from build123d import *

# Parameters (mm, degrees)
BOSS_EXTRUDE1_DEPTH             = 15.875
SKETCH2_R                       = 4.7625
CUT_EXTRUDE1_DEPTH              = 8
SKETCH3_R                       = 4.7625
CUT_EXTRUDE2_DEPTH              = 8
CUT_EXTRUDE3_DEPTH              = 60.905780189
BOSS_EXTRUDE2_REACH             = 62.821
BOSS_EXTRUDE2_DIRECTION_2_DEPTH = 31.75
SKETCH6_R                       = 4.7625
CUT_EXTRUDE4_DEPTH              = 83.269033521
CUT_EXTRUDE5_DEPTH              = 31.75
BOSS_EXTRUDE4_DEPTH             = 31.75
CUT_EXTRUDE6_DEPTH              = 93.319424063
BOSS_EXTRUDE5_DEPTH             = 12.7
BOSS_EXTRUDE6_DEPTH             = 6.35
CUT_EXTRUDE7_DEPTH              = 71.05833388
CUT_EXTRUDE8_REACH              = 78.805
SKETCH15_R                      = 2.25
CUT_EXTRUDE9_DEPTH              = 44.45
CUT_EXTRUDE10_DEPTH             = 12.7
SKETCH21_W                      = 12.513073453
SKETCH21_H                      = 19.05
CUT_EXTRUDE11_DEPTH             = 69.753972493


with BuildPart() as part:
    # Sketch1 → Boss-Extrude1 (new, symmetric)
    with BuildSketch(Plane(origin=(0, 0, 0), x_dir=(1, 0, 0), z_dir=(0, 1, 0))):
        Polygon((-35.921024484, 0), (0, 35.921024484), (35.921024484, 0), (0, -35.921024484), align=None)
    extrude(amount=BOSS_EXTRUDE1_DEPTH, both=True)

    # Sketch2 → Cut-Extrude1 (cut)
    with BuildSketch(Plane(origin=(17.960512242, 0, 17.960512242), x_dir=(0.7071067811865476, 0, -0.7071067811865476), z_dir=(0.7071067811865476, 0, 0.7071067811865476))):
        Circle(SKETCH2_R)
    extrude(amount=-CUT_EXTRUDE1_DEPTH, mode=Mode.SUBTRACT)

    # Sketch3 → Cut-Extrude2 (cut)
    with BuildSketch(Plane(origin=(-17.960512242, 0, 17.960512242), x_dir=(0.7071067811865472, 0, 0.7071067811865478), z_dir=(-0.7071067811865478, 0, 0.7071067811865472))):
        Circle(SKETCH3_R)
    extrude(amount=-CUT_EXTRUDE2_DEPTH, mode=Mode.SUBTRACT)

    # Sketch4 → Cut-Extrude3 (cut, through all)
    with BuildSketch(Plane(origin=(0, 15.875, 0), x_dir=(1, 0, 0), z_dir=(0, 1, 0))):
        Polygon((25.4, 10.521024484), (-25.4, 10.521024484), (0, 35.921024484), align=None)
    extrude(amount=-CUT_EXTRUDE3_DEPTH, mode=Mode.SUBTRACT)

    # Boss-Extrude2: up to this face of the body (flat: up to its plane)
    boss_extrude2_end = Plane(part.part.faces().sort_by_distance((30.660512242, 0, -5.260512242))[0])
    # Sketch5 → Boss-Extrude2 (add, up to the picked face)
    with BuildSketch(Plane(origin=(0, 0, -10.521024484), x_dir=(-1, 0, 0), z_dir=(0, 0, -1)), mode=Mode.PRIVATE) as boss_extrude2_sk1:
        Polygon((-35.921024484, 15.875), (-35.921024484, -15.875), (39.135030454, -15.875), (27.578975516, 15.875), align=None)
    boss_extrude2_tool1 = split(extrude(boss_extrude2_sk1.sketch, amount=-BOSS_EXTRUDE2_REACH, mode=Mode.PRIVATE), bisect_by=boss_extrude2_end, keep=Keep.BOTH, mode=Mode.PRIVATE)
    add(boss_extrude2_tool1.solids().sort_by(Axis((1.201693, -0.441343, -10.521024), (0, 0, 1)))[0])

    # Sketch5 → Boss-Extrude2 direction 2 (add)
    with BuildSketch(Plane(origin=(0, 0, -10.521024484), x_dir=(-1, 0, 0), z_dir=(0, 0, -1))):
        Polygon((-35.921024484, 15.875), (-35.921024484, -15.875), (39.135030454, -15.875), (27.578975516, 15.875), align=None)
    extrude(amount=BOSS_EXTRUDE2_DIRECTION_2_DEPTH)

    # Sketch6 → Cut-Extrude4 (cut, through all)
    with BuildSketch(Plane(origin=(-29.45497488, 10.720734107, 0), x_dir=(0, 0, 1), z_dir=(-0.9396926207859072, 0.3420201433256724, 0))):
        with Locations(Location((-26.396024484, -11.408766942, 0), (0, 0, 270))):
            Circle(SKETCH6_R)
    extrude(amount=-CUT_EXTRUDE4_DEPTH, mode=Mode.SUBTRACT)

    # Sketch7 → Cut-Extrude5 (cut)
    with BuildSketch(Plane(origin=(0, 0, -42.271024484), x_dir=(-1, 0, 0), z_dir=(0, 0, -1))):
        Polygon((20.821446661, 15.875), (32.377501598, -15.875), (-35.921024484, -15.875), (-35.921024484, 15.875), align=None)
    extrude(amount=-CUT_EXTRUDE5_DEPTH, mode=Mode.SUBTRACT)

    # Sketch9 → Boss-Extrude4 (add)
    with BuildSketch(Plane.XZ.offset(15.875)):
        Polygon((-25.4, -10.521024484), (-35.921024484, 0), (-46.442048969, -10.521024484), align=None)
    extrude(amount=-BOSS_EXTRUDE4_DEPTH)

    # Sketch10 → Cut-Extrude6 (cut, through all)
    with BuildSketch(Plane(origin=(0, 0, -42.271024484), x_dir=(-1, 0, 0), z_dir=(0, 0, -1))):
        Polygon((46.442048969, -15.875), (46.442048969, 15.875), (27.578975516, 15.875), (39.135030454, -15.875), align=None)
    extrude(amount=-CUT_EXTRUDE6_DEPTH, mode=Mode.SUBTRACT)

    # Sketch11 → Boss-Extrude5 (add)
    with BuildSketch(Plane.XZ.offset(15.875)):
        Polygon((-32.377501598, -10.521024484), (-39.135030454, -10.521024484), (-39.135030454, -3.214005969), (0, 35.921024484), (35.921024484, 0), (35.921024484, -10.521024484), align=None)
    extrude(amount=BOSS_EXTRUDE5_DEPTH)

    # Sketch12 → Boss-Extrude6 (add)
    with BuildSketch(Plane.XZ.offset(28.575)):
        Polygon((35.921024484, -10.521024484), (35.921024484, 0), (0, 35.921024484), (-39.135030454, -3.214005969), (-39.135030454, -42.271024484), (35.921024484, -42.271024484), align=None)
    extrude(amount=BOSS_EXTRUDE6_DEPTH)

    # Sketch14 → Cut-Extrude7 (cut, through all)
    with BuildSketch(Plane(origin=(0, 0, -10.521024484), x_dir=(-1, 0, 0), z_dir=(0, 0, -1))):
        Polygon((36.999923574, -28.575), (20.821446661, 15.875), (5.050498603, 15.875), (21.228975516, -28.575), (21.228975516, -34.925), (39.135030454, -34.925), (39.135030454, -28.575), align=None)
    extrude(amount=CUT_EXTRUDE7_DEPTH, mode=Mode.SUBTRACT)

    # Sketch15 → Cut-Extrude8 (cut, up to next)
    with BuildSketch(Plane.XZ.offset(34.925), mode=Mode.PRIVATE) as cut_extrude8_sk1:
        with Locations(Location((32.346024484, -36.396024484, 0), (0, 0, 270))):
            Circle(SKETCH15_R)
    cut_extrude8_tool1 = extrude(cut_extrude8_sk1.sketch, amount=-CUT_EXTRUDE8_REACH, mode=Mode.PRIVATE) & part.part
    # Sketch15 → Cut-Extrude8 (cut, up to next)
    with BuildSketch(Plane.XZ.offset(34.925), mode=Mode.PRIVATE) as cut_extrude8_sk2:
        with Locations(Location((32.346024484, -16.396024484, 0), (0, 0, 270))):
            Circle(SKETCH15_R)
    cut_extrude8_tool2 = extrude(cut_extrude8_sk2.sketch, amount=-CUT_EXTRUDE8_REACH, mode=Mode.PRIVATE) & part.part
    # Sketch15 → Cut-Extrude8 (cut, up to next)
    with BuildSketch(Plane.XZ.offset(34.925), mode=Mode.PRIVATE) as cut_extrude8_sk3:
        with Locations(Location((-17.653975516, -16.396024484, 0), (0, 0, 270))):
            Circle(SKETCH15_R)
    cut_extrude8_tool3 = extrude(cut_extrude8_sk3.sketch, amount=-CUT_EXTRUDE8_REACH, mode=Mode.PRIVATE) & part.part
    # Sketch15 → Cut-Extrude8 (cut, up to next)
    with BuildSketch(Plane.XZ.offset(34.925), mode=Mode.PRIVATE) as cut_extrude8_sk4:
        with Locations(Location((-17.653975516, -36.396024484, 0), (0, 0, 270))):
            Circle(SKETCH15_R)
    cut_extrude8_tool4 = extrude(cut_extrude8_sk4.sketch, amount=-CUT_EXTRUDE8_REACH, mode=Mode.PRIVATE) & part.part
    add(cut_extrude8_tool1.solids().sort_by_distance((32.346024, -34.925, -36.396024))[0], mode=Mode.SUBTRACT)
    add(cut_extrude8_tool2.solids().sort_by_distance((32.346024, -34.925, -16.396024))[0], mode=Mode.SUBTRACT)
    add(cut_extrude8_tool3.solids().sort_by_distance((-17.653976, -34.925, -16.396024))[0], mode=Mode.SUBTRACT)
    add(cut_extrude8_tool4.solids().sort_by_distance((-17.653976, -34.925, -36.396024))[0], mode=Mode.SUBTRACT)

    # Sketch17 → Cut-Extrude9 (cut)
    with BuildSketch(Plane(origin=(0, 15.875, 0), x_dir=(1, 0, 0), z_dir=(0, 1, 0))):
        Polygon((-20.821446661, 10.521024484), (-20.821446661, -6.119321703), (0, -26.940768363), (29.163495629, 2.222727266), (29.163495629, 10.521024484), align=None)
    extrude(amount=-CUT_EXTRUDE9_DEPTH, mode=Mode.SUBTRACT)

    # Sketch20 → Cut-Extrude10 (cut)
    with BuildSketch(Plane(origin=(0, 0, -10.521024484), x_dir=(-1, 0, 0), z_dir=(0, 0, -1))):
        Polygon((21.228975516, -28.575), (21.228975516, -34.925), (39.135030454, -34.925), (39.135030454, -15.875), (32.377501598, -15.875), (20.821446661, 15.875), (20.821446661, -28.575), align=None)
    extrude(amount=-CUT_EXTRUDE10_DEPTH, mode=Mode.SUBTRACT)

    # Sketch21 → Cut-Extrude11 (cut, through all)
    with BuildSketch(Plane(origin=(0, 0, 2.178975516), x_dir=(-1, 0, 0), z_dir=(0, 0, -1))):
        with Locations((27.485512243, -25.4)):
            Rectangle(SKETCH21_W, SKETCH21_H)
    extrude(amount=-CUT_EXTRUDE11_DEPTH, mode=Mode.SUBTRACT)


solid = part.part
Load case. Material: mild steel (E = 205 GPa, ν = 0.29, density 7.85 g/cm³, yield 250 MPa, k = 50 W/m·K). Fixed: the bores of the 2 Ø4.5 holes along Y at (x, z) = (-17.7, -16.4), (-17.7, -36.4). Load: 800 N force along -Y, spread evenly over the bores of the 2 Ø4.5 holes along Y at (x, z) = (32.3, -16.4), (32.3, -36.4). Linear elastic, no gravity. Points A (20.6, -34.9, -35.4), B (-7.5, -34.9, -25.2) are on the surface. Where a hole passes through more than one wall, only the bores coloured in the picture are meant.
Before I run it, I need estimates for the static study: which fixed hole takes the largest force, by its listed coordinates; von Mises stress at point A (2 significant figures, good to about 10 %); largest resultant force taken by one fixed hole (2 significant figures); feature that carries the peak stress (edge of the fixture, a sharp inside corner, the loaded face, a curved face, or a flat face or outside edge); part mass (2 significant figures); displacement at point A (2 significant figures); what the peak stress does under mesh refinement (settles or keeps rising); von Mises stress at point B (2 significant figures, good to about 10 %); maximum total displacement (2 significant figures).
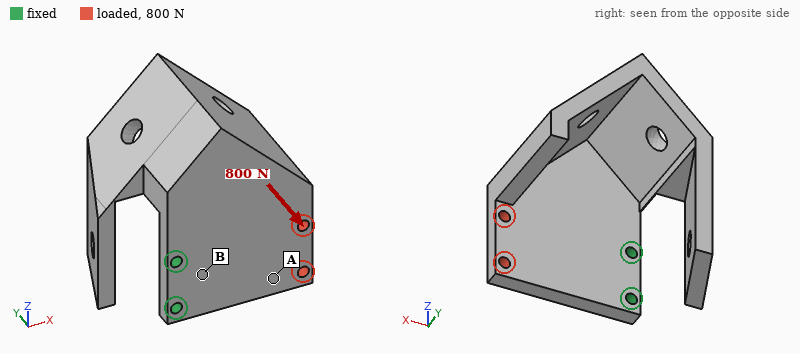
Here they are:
(-17.7, -16.4)
31 MPa
510 N
edge of the fixture
450 g
0.11 mm
keeps rising
91 MPa
0.24 mm
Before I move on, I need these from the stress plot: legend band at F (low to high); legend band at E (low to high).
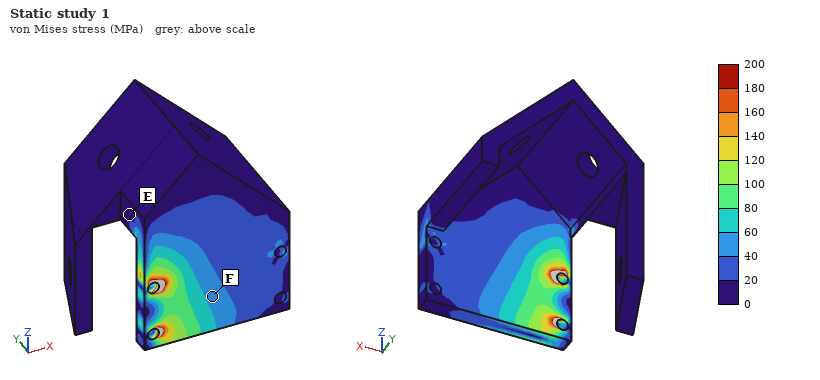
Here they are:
40 to 60 MPa
0 to 20 MPa
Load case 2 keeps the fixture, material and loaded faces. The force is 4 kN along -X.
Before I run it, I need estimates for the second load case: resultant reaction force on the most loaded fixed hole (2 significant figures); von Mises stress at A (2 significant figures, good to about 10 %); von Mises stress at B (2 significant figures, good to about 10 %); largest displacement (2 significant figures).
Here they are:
2.0 kN
21 MPa
13 MPa
7.8 µm
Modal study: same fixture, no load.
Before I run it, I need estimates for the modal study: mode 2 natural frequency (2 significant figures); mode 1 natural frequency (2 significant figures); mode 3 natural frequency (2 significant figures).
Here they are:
670 Hz
550 Hz
1100 Hz
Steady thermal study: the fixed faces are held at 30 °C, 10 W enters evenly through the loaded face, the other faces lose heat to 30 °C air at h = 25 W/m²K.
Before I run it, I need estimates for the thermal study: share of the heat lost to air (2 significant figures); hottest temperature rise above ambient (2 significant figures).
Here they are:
43 %
34 K
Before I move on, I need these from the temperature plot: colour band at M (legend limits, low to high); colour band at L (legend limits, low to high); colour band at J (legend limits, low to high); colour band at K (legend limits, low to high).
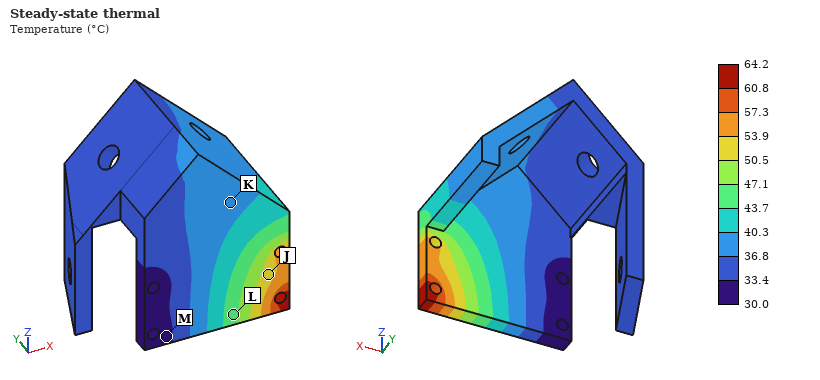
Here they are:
30.0 to 33.4 °C
43.7 to 47.1 °C
50.5 to 53.9 °C
36.8 to 40.3 °C
